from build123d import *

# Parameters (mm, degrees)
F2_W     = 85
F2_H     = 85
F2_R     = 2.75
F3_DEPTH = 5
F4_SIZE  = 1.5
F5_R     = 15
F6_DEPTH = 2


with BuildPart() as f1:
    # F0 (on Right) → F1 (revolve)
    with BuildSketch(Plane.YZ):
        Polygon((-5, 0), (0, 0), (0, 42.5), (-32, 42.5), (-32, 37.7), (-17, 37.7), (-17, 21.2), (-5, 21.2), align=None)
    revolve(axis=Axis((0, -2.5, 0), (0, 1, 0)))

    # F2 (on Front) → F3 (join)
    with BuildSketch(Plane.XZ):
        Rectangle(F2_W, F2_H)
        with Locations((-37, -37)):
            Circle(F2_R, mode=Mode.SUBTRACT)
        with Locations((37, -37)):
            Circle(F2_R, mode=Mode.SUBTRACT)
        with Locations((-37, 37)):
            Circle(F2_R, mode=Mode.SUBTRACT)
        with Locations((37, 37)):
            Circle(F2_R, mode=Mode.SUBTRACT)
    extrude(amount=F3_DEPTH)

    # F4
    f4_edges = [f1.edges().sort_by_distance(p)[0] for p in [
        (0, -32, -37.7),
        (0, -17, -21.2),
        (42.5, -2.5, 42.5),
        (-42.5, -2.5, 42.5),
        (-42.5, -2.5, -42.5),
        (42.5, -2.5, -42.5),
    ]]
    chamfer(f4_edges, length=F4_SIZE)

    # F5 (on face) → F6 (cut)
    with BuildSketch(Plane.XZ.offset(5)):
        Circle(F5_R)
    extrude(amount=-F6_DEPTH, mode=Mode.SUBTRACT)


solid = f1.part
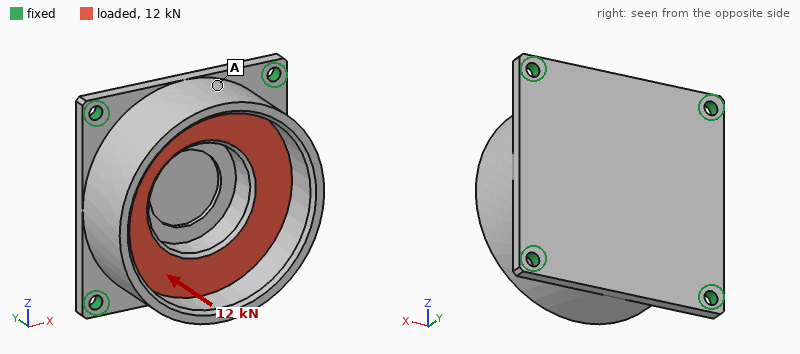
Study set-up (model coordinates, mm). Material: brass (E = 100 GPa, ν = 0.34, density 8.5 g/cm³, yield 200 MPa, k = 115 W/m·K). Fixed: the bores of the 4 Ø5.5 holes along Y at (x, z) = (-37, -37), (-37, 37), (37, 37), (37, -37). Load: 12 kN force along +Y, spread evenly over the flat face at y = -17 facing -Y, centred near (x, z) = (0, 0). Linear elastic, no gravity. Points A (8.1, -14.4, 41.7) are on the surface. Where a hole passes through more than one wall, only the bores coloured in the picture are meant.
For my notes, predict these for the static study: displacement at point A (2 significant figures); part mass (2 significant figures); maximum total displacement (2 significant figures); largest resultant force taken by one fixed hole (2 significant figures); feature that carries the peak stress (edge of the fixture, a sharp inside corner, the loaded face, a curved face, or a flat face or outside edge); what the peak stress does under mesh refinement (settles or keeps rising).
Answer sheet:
34 µm
880 g
43 µm
3.5 kN
edge of the fixture
keeps rising
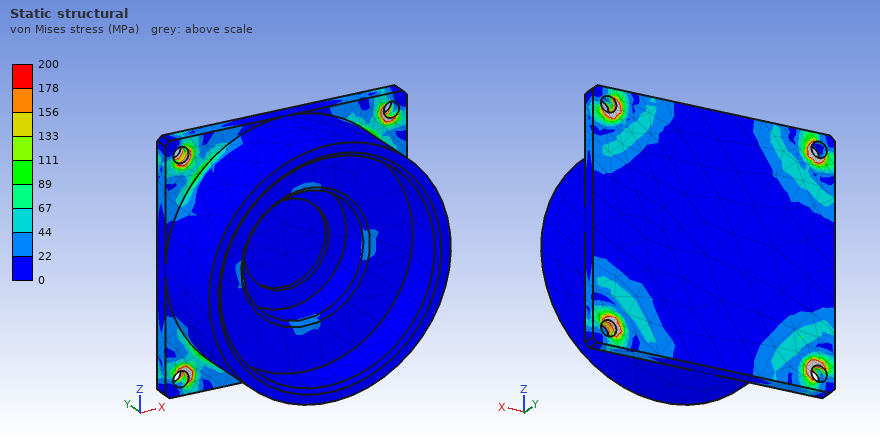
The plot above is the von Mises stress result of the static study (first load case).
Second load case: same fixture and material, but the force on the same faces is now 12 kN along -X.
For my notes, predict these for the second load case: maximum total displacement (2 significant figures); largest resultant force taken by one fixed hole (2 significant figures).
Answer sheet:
28 µm
3.5 kN
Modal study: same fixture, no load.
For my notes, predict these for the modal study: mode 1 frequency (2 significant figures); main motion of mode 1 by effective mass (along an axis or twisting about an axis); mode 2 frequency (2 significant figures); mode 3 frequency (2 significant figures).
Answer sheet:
3200 Hz
along Y
4000 Hz
4000 Hz
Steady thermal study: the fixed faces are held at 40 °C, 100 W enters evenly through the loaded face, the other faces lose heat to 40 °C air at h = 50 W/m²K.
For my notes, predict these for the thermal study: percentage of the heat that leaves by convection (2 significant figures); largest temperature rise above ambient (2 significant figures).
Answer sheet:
25 %
25 K
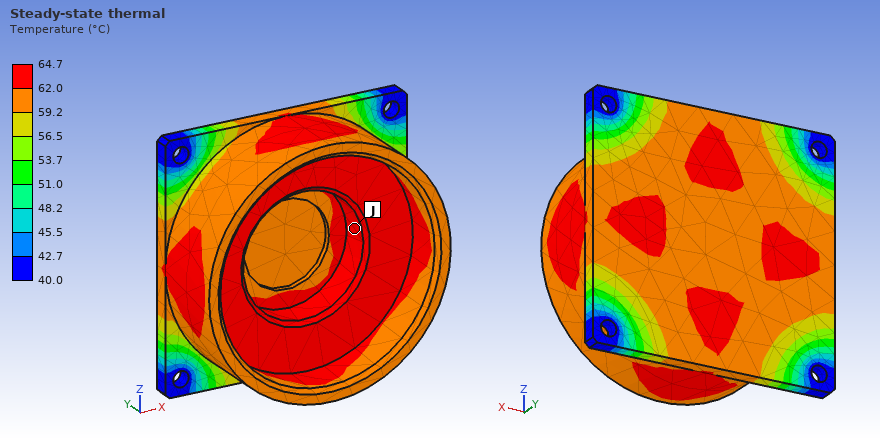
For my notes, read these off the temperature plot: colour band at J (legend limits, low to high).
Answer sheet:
62.0 to 64.7 °C
